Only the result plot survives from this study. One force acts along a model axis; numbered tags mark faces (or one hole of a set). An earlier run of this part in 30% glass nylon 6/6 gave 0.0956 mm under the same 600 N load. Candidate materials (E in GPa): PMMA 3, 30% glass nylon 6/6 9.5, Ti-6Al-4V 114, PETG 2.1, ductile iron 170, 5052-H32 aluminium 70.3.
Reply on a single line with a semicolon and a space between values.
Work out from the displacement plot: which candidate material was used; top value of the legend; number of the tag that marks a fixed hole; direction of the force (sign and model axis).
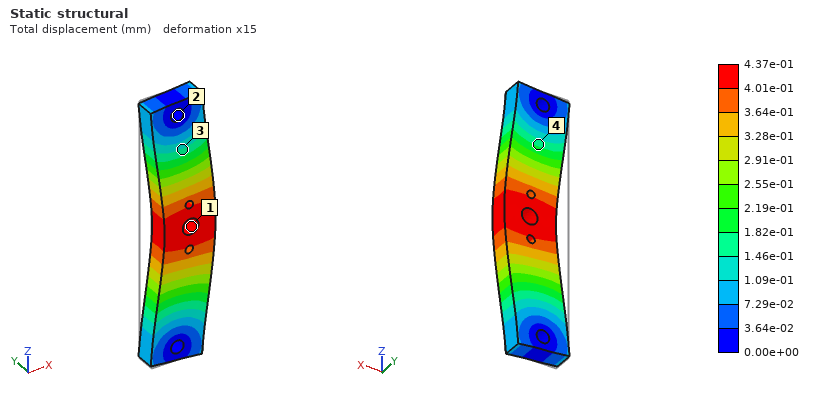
PETG; 4.37e-01 mm; 2; +X
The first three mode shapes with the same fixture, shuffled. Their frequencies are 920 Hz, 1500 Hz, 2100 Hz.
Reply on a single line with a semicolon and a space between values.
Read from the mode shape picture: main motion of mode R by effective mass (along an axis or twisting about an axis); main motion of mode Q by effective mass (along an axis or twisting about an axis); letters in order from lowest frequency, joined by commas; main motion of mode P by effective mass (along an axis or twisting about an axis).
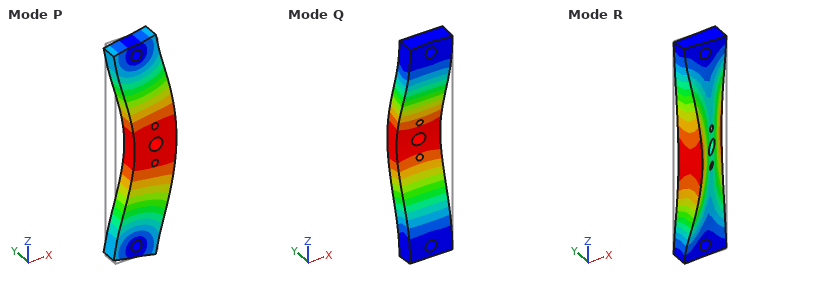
twisting about Z; along Y; Q, P, R; along X
